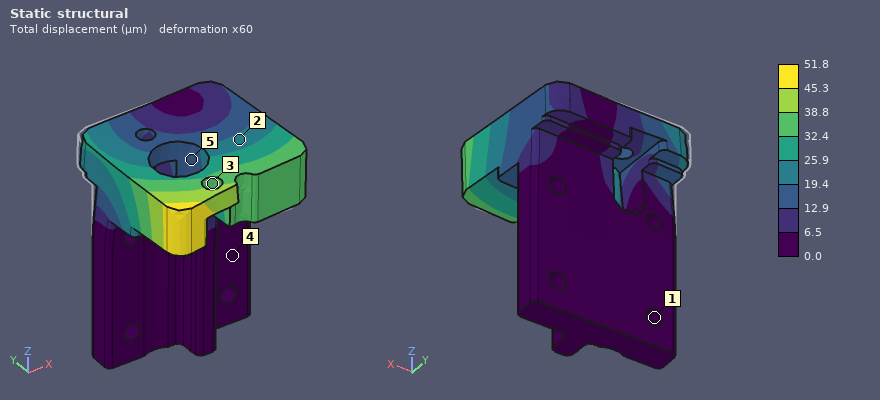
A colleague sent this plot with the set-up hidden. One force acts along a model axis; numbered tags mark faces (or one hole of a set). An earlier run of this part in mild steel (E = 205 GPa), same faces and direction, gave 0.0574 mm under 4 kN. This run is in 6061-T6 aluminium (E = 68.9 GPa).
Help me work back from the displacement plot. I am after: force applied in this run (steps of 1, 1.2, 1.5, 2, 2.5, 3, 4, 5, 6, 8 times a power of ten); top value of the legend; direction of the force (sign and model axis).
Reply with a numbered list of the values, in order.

1. 1.2 kN
2. 51.8 µm
3. +X
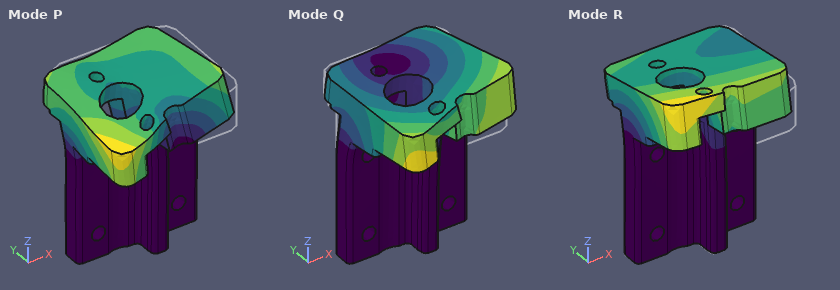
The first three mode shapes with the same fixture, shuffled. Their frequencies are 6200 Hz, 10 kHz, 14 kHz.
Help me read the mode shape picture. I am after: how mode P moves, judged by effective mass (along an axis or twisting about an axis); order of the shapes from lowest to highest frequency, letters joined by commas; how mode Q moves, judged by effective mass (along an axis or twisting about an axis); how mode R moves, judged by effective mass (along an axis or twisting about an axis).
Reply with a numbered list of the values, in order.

1. along X
2. R, Q, P
3. along X
4. along Y
